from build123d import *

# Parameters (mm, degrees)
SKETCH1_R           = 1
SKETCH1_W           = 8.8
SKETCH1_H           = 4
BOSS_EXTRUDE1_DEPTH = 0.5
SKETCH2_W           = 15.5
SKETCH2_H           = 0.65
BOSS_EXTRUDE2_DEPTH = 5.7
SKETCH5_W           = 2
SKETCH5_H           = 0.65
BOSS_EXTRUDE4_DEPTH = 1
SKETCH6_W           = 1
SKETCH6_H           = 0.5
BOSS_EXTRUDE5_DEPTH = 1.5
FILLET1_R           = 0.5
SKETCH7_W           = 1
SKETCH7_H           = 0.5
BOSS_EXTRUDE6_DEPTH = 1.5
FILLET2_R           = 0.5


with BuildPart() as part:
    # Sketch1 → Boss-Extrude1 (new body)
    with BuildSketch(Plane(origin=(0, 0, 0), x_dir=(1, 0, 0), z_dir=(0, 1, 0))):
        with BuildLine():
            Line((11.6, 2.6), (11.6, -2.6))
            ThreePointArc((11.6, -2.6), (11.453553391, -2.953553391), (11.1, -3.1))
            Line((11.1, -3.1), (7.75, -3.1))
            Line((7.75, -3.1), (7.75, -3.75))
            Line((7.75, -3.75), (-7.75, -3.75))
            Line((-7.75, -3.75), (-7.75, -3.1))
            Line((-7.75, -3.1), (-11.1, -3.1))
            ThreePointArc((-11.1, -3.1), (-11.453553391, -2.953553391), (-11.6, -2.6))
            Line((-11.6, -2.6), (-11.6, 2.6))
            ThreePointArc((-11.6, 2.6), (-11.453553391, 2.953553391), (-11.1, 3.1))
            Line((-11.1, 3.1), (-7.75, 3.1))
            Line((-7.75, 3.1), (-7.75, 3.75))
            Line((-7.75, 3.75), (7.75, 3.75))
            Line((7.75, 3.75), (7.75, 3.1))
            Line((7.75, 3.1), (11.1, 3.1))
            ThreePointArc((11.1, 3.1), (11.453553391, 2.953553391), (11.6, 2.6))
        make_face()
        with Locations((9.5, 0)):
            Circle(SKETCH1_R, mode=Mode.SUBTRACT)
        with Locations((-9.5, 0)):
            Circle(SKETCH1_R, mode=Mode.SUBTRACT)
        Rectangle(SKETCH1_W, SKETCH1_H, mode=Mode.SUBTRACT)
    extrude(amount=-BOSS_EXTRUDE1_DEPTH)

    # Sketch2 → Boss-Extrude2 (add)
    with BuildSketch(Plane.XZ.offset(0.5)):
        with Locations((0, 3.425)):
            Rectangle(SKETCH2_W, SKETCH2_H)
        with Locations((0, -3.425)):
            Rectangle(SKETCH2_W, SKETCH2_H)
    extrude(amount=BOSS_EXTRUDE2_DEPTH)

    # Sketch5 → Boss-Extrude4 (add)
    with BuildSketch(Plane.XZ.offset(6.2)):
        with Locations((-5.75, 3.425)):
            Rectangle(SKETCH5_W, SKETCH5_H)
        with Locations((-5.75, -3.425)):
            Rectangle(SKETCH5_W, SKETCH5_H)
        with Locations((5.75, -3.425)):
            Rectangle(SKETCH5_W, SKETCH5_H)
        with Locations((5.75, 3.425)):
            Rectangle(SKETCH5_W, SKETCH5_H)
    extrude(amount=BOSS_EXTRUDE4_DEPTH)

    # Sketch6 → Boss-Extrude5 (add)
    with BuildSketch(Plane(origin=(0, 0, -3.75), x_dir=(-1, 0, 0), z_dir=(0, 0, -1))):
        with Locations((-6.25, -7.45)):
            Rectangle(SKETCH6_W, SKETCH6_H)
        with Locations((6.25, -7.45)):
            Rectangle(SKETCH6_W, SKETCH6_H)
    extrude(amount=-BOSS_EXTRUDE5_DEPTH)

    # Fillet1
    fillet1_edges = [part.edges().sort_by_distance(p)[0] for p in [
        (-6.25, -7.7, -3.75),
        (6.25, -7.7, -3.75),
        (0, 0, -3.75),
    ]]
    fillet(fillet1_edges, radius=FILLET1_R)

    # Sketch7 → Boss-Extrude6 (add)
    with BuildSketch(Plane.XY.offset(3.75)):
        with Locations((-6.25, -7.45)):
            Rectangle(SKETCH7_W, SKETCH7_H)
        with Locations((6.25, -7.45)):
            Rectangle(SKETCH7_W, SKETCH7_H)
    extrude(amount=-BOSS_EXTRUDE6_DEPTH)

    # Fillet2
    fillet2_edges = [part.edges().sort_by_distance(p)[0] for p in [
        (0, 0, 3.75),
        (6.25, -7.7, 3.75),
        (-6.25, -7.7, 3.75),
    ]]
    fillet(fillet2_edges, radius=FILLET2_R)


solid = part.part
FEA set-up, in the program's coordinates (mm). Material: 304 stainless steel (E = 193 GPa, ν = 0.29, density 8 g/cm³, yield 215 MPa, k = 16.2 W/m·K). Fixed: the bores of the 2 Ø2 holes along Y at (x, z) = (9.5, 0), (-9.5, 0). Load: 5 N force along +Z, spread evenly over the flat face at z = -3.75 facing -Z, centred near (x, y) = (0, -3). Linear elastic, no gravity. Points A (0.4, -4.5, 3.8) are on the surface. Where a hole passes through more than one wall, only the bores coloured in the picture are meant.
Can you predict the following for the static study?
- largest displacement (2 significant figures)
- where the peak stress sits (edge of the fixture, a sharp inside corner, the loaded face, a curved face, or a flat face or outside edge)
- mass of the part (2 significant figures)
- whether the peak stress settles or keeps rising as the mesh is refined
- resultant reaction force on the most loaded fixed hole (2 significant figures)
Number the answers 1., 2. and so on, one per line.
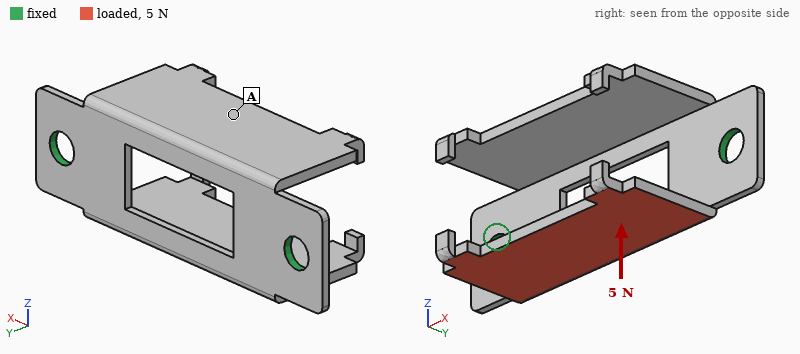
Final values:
1. 22 µm
2. a sharp inside corner
3. 1.5 g
4. keeps rising
5. 2.6 N
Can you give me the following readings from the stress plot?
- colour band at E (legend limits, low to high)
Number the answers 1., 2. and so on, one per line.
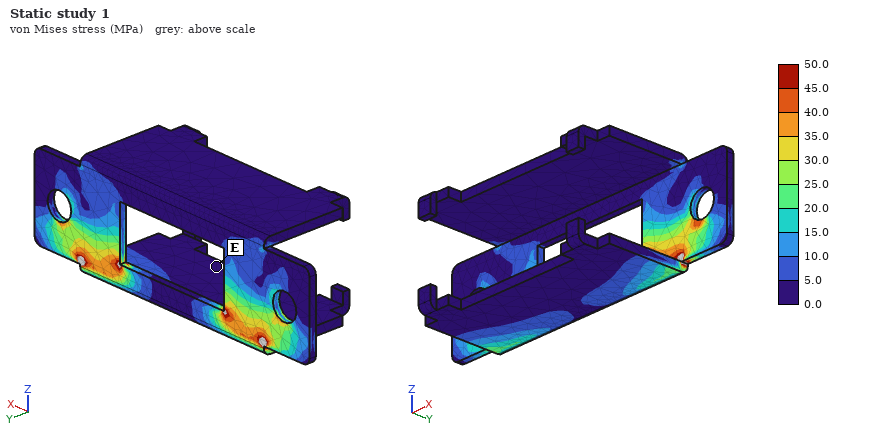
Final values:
1. 0.0 to 5.0 MPa
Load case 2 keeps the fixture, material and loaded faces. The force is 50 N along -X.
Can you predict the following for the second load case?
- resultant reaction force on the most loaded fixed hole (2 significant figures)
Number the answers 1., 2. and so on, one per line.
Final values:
1. 28 N
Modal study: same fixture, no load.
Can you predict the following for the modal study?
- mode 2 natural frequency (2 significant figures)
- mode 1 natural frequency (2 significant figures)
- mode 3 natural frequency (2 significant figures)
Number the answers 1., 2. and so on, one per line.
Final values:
1. 4200 Hz
2. 4200 Hz
3. 10 kHz
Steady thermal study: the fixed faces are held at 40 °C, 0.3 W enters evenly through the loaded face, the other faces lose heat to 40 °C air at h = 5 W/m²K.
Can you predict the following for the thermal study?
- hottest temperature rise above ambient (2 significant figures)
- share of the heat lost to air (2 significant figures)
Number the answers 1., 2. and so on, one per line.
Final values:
1. 25 K
2. 8.7 %
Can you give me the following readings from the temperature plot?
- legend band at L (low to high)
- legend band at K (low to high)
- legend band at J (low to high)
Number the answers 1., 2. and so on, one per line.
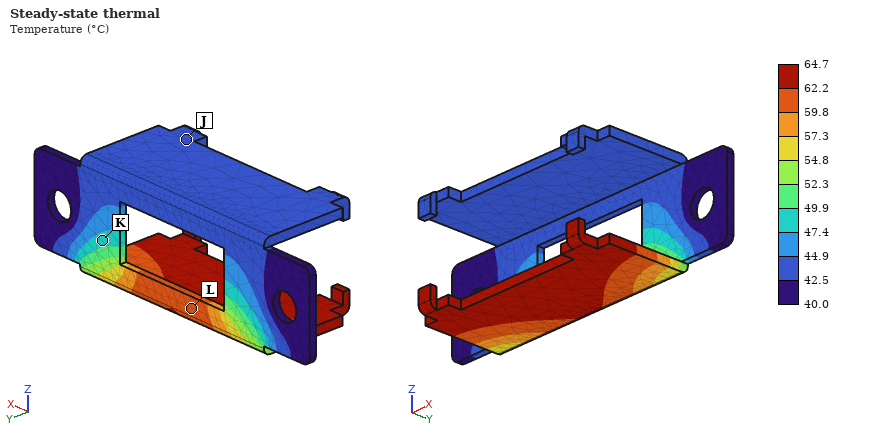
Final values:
1. 59.8 to 62.2 °C
2. 47.4 to 49.9 °C
3. 42.5 to 44.9 °C
